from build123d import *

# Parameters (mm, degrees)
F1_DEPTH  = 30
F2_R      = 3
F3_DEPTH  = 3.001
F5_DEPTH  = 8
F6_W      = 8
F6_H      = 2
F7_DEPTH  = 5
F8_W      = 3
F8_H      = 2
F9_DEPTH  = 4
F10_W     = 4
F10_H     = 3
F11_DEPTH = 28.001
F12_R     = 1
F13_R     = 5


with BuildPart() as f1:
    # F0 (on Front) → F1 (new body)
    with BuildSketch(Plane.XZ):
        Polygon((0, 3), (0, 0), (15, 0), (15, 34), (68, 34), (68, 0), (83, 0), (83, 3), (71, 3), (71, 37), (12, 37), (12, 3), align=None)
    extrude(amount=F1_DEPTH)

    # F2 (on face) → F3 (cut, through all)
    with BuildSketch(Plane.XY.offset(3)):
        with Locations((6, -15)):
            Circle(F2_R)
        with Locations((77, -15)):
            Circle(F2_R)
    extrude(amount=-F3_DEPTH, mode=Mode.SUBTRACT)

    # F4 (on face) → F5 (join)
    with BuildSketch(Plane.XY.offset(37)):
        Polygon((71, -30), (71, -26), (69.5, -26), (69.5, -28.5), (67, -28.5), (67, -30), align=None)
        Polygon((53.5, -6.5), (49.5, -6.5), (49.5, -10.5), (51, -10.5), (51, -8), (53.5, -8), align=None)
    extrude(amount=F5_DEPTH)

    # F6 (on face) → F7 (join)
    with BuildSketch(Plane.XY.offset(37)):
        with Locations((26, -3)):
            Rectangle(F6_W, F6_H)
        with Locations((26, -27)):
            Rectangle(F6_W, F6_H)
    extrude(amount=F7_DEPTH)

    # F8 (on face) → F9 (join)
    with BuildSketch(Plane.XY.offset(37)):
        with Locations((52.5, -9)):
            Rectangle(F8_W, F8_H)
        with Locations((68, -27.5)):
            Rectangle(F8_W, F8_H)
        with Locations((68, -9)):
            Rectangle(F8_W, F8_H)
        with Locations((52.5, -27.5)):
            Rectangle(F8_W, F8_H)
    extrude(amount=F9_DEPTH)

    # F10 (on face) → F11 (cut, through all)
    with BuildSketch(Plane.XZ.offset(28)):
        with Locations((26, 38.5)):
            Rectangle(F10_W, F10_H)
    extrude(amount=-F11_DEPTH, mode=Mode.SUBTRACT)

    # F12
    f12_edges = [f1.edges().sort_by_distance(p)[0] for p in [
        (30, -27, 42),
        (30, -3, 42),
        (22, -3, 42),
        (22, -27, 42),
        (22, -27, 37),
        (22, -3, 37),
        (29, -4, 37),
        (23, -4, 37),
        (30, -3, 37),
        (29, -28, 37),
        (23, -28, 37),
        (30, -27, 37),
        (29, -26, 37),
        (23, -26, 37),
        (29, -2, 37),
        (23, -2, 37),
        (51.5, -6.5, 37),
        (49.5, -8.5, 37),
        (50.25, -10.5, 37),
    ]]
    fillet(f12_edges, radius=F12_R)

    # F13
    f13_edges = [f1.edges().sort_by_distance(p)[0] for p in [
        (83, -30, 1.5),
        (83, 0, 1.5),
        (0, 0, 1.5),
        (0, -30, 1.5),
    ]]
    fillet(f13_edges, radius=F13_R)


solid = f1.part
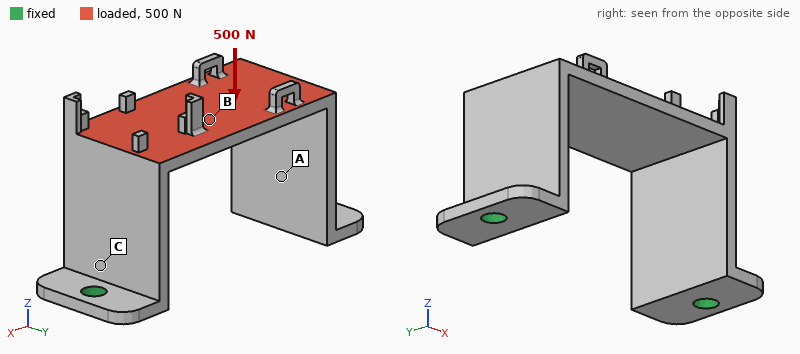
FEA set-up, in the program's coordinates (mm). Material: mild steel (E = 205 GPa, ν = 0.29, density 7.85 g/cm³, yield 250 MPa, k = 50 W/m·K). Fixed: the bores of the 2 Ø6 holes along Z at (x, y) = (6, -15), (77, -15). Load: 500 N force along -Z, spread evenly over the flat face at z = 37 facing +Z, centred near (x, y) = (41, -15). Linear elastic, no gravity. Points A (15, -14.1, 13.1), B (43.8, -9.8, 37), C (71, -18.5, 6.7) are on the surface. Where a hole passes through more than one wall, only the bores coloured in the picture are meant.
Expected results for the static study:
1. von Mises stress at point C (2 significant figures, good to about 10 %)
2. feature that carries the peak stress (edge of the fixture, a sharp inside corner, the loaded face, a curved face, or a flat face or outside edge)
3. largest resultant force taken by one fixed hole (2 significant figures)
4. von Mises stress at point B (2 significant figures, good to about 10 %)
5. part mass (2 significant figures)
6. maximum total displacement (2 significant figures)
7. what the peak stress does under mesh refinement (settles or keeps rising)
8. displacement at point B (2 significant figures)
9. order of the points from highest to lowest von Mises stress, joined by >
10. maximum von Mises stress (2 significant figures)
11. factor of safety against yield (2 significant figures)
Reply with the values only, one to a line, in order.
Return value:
15 MPa
the loaded face
260 N
33 MPa
110 g
30 µm
settles
28 µm
B > C > A
45 MPa
5.5
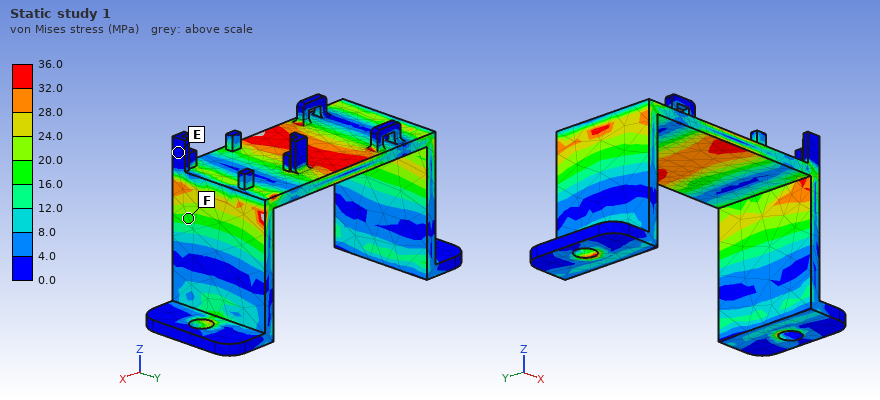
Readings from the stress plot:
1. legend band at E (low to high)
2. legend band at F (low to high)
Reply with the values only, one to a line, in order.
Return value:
0.0 to 4.0 MPa
16.0 to 20.0 MPa
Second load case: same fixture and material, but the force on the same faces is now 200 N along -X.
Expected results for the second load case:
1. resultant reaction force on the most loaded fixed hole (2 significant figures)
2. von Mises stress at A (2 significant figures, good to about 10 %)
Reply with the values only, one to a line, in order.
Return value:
120 N
11 MPa
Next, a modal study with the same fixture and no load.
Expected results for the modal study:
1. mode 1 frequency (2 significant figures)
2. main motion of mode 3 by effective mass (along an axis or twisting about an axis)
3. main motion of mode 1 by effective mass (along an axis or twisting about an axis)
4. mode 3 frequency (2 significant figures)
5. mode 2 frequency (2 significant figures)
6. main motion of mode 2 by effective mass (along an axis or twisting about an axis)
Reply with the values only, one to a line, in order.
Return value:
1300 Hz
twisting about Z
along X
2400 Hz
1600 Hz
along Y
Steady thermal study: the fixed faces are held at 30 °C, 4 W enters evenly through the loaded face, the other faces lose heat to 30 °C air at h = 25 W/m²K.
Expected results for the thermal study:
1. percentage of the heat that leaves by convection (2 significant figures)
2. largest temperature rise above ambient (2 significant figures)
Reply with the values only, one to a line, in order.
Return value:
43 %
16 K
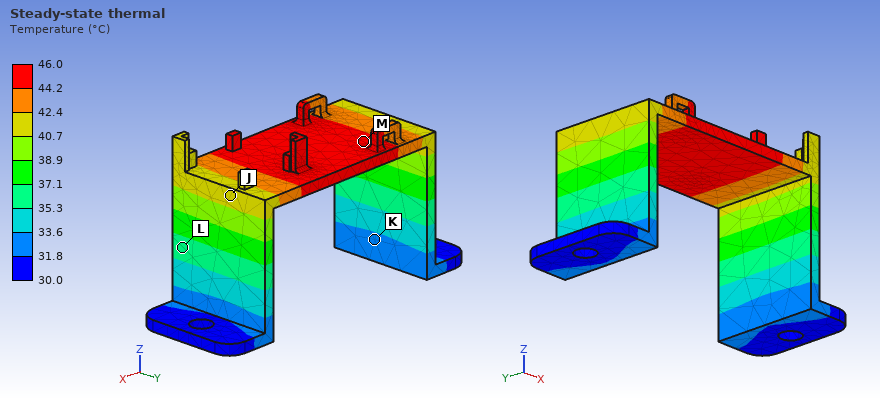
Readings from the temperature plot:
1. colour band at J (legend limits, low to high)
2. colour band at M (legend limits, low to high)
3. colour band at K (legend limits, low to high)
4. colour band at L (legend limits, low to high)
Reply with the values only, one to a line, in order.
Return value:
40.7 to 42.4 °C
44.2 to 46.0 °C
31.8 to 33.6 °C
35.3 to 37.1 °C
